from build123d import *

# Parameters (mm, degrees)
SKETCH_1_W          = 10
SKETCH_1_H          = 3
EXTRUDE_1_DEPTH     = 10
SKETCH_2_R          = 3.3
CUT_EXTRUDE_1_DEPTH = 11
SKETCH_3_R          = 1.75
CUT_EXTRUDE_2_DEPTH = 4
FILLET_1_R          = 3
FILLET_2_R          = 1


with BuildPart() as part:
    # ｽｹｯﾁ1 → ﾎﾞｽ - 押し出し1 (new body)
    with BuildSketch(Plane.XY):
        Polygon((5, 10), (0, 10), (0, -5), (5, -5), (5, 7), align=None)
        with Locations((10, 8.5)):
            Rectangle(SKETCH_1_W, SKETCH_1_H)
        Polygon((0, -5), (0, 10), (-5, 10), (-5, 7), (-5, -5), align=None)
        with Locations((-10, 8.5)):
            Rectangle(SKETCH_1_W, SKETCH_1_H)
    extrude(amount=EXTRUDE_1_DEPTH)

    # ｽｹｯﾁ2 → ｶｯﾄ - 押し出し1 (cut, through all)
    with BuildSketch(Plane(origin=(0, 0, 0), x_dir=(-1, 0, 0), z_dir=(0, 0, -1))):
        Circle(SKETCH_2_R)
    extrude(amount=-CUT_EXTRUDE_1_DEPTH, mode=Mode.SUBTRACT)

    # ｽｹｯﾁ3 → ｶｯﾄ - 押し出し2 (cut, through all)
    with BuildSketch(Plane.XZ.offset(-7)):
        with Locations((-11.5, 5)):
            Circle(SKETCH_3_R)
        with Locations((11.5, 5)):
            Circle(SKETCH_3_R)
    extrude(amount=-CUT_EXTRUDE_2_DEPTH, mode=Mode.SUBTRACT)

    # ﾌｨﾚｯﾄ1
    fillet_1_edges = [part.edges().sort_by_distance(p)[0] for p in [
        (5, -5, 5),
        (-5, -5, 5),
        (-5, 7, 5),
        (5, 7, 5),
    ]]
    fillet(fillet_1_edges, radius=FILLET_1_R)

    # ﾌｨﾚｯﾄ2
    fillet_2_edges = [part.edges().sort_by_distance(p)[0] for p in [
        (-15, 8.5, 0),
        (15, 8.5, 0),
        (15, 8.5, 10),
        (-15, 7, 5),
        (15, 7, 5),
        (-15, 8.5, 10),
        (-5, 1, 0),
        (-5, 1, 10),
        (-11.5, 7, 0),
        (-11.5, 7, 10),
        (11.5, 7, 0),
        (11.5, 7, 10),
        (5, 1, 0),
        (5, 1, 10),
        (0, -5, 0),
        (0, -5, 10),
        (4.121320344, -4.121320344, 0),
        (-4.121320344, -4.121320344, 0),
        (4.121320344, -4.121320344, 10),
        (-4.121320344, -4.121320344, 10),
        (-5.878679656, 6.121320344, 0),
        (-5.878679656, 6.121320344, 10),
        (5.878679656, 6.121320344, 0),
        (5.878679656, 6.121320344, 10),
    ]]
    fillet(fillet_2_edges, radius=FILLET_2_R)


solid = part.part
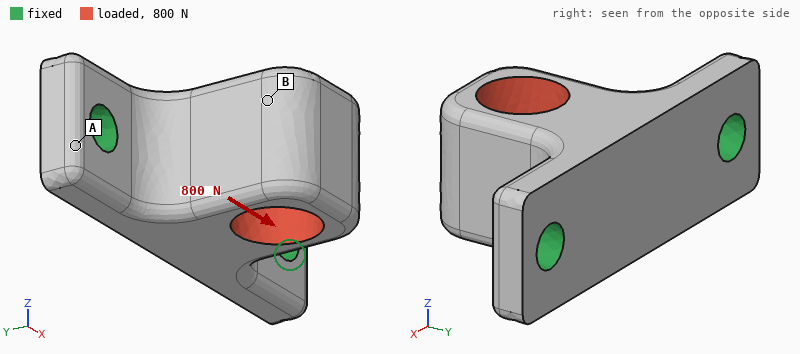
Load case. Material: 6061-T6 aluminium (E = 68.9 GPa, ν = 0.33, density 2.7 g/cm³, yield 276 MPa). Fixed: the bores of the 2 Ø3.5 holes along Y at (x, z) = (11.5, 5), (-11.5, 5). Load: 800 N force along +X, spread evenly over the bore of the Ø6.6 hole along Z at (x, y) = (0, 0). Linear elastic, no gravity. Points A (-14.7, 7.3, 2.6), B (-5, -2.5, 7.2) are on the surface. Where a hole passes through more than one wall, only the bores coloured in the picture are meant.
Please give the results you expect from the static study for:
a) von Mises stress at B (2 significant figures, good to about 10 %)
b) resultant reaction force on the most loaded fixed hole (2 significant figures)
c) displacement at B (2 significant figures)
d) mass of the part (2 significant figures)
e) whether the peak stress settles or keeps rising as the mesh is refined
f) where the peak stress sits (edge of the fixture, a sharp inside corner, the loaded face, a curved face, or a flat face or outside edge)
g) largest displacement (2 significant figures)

24 MPa
560 N
26 µm
4.5 g
keeps rising
edge of the fixture
29 µm
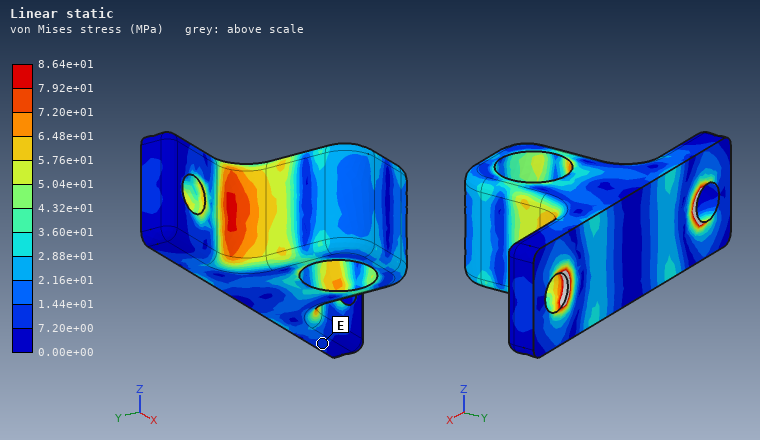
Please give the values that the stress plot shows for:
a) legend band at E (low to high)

7.20e+00 to 1.44e+01 MPa
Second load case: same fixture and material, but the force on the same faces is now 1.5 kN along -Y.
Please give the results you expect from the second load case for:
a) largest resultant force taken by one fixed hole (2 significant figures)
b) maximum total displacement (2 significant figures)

850 N
22 µm
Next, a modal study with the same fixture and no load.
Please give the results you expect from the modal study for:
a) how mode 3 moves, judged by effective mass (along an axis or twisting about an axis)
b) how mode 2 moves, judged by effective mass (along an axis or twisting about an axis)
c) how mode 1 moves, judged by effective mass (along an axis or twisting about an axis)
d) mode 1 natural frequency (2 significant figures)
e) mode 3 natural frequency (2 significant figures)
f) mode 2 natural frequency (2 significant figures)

along Y
along X
along Z
12 kHz
26 kHz
24 kHz
